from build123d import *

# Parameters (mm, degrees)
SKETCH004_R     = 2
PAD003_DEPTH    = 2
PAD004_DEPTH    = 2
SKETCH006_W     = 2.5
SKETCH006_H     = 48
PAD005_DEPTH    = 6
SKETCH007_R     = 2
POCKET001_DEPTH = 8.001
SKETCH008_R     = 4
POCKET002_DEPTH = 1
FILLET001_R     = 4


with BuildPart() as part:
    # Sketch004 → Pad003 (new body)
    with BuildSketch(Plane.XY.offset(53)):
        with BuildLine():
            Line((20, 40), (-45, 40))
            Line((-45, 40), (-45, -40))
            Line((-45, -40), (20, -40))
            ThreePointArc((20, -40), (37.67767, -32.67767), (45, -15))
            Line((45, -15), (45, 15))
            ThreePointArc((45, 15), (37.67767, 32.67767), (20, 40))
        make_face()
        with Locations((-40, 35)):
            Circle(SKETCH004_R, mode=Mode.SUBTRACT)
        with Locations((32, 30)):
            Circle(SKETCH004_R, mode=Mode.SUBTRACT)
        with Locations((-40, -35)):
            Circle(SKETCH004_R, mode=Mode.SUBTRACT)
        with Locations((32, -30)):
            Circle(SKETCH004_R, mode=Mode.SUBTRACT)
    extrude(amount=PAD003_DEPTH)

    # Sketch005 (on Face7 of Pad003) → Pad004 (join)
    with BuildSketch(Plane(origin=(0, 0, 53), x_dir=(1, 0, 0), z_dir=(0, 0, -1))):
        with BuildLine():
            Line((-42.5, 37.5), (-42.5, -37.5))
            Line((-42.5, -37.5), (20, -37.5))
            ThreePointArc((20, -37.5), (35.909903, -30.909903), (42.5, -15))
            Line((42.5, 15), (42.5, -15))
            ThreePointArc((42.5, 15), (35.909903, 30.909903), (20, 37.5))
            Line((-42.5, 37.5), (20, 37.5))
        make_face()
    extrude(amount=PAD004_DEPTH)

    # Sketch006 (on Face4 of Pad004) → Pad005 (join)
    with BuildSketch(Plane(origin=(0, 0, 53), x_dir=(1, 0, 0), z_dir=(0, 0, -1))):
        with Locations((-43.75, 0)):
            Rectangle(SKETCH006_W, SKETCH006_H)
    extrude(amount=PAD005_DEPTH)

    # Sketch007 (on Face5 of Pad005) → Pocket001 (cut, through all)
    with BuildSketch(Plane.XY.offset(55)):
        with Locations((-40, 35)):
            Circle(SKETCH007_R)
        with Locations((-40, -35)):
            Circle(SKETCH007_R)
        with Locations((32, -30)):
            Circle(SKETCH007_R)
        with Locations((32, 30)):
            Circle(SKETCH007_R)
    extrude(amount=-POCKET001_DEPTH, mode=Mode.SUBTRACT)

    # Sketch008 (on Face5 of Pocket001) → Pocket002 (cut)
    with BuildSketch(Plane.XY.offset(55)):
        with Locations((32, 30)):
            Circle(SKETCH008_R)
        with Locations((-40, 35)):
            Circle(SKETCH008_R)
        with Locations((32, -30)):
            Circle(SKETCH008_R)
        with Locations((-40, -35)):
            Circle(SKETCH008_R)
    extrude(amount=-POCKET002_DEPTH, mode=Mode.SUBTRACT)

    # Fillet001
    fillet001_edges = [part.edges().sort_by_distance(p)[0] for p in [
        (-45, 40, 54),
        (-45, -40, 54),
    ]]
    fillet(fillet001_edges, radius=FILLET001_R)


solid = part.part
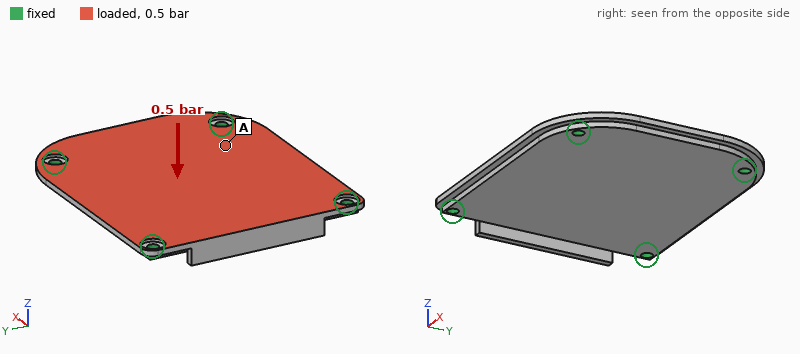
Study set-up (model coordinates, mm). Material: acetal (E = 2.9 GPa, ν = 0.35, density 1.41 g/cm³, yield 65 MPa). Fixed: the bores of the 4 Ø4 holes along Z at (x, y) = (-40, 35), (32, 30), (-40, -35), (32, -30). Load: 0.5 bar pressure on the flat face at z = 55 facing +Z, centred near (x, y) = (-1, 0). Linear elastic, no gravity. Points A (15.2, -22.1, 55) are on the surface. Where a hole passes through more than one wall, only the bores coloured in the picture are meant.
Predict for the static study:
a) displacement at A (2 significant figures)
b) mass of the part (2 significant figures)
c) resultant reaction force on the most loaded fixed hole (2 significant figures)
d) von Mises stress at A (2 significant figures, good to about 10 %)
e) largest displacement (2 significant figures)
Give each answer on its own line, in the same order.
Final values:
0.32 mm
37 g
110 N
3.0 MPa
0.60 mm
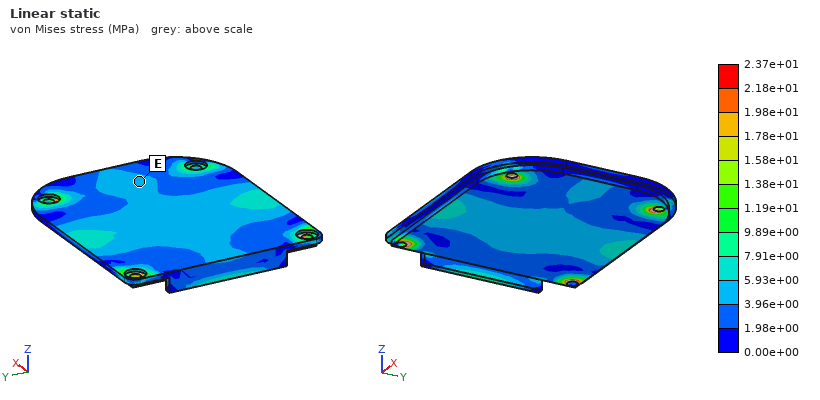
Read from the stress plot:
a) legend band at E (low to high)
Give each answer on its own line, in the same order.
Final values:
3.96e+00 to 5.93e+00 MPa
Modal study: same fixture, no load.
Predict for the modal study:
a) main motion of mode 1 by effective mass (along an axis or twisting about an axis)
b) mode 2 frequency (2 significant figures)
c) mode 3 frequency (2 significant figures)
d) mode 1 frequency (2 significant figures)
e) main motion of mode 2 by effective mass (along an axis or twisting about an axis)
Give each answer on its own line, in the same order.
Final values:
along Z
1200 Hz
1300 Hz
730 Hz
twisting about X
